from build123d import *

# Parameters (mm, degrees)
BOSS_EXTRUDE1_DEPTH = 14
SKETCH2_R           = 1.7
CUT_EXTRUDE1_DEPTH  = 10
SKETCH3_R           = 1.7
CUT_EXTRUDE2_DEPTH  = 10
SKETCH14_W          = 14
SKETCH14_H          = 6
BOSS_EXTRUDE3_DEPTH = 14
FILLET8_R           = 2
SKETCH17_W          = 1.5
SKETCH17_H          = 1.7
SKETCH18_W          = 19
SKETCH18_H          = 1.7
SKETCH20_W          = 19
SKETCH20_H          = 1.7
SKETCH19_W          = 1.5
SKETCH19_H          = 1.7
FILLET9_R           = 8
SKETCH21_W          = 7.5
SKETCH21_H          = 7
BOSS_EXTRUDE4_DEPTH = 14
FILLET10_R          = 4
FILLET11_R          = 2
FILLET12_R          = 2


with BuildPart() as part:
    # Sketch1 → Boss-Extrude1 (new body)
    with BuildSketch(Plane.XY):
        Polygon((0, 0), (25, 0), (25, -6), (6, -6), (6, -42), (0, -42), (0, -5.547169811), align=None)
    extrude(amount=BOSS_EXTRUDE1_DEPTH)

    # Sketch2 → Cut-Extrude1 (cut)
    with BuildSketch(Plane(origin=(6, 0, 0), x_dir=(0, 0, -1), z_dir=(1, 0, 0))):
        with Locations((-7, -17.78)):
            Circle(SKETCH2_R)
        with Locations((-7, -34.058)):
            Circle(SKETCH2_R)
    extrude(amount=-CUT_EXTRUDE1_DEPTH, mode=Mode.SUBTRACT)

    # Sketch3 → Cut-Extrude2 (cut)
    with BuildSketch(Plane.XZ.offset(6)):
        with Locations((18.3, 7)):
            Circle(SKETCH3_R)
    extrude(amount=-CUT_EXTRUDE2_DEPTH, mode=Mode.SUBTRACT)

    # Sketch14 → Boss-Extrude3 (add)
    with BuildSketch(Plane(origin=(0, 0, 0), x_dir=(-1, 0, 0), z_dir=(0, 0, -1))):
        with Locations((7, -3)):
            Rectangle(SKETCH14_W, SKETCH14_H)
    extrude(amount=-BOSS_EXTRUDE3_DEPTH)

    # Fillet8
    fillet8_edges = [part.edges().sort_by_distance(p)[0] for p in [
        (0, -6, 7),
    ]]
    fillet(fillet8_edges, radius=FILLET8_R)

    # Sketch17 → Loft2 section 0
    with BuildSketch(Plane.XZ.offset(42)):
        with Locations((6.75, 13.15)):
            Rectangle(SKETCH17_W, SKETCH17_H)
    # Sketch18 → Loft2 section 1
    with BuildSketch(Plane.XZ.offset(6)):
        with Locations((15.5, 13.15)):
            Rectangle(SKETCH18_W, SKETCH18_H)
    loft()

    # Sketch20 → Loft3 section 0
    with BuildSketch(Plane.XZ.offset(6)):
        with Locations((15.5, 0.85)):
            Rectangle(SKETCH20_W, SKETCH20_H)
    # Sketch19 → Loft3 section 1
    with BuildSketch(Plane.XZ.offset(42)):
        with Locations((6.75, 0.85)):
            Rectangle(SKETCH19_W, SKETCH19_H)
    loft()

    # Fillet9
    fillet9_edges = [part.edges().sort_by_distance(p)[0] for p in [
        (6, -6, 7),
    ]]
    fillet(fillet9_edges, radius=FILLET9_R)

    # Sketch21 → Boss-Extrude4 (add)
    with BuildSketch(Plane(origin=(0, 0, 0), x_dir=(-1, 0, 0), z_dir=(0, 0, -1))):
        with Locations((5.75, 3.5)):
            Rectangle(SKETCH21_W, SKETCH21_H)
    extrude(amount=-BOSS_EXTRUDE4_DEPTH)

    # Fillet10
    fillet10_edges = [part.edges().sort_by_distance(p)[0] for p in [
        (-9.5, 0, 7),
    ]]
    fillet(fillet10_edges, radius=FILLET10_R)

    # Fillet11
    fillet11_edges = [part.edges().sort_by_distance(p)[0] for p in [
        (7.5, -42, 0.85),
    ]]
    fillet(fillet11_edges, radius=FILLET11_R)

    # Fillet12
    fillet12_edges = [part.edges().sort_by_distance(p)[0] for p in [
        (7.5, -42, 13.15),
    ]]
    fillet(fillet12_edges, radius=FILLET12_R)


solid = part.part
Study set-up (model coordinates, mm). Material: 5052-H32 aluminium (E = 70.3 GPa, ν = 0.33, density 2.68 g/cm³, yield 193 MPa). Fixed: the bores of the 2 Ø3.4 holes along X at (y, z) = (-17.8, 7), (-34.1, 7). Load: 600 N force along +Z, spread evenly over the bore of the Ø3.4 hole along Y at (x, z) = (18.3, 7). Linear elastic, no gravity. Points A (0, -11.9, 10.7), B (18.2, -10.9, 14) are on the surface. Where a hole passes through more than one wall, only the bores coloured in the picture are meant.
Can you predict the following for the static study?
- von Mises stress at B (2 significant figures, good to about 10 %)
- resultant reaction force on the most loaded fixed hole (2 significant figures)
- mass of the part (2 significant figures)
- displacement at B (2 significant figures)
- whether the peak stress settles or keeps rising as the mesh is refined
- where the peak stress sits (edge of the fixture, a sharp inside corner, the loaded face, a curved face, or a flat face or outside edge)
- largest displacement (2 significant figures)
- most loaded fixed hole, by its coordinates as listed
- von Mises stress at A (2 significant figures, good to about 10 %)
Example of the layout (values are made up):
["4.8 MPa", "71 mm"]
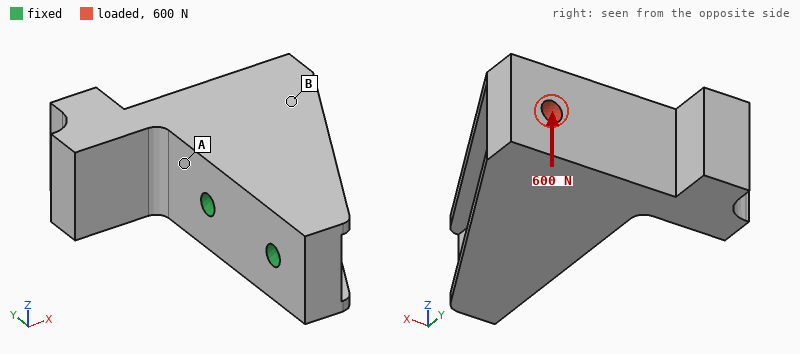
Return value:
["12 MPa", "960 N", "22 g", "56 µm", "keeps rising", "edge of the fixture", "83 µm", "(-17.8, 7)", "28 MPa"]
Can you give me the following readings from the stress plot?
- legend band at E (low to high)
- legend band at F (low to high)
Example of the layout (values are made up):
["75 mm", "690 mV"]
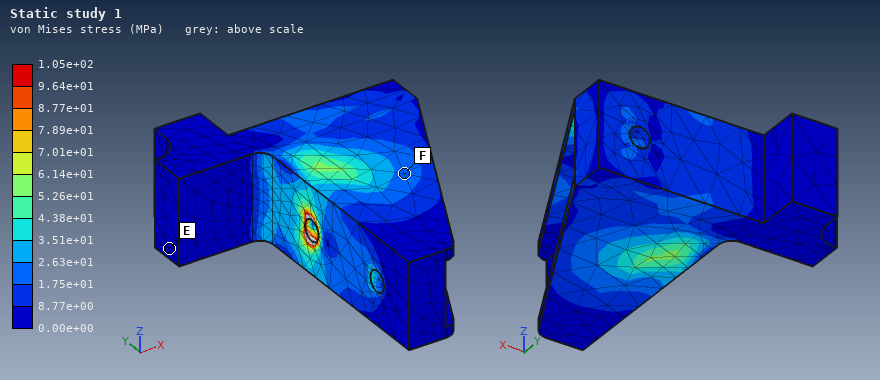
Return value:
["0.00e+00 to 8.77e+00 MPa", "1.75e+01 to 2.63e+01 MPa"]
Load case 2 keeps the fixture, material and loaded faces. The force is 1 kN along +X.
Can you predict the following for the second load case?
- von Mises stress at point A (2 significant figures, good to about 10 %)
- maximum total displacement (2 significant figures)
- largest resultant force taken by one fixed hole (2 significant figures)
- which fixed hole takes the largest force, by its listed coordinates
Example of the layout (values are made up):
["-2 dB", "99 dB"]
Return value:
["20 MPa", "42 µm", "1.5 kN", "(-17.8, 7)"]
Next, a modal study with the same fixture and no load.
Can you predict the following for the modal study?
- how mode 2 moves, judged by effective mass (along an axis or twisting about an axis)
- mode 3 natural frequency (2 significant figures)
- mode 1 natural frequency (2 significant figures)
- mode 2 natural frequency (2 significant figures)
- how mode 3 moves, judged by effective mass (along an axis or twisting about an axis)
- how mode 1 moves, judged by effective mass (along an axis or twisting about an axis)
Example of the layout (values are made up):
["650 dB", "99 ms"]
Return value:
["along X", "8300 Hz", "6400 Hz", "7000 Hz", "along Z", "twisting about Y"]
